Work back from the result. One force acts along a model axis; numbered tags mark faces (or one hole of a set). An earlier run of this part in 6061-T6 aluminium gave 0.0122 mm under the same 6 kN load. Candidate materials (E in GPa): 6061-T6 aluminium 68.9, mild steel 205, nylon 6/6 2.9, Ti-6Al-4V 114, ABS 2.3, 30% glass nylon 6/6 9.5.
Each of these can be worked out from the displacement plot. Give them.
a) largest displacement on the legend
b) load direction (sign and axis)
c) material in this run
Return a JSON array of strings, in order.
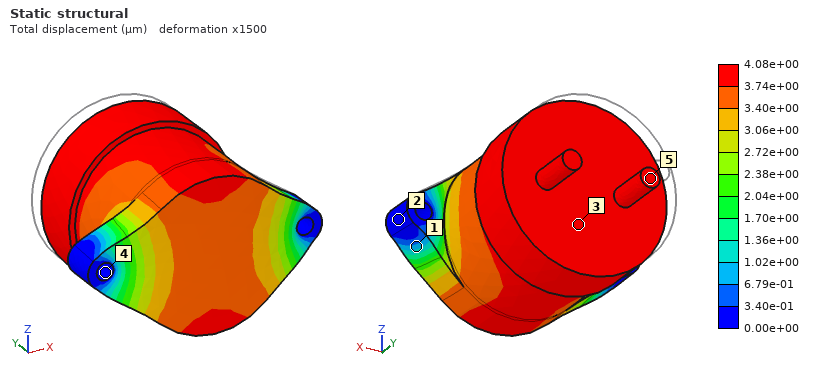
["4.08e+00 µm", "-Y", "mild steel"]
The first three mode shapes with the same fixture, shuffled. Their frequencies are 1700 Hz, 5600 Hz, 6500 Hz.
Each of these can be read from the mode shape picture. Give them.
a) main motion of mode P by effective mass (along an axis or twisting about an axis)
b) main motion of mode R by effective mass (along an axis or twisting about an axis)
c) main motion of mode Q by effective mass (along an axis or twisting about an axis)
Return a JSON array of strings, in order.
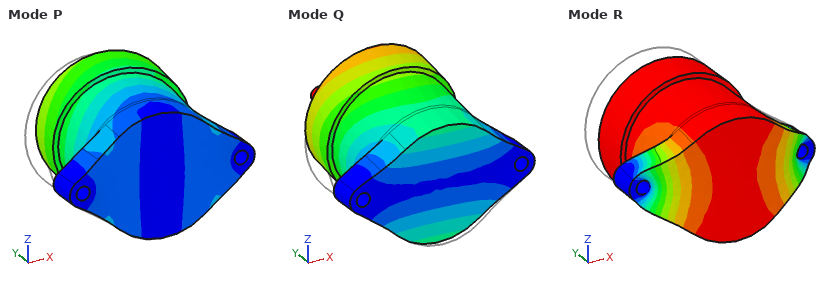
["along X", "along Y", "along Z"]
